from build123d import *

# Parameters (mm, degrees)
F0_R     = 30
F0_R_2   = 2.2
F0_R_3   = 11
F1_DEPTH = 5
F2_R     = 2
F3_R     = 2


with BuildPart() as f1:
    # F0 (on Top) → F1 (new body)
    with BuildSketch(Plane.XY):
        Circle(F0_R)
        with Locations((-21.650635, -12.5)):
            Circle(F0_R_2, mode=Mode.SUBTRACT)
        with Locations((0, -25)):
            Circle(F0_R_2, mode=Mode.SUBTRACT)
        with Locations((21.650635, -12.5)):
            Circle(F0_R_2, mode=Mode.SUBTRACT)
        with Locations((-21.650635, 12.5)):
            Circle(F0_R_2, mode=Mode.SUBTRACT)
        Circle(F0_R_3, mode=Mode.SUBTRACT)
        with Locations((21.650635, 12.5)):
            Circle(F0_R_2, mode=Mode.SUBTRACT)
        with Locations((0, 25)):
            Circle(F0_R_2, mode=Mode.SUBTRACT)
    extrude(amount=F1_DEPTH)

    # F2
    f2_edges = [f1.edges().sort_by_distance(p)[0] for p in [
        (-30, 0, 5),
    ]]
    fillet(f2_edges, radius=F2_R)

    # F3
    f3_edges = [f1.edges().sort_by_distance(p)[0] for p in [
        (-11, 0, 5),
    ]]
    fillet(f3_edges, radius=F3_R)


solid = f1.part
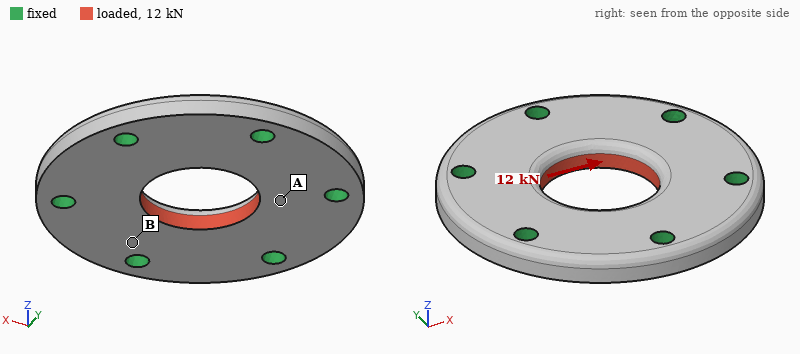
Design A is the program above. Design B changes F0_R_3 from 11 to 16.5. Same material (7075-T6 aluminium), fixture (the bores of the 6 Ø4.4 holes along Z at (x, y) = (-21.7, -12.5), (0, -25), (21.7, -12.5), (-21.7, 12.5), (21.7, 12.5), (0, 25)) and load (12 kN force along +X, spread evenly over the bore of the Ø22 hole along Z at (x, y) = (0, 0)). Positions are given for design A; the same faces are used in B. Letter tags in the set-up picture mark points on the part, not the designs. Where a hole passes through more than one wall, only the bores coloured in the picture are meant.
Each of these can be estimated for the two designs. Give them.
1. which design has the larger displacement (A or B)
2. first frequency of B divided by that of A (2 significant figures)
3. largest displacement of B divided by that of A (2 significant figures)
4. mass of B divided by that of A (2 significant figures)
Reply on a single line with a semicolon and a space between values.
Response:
A; 1.5; 0.84; 0.79
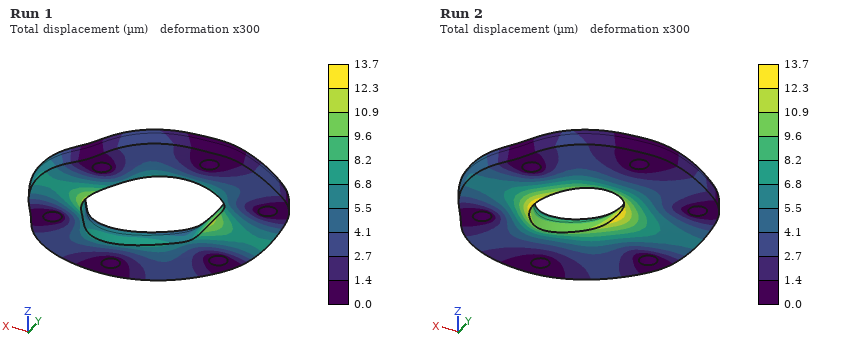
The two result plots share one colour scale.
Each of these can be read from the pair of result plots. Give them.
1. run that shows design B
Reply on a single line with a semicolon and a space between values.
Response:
Run 1
